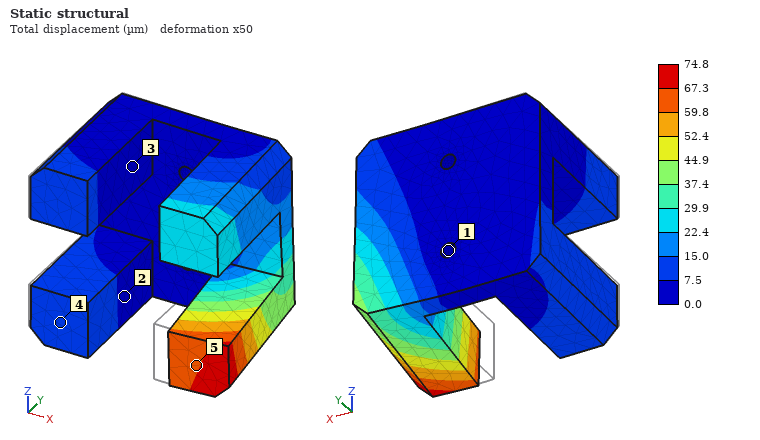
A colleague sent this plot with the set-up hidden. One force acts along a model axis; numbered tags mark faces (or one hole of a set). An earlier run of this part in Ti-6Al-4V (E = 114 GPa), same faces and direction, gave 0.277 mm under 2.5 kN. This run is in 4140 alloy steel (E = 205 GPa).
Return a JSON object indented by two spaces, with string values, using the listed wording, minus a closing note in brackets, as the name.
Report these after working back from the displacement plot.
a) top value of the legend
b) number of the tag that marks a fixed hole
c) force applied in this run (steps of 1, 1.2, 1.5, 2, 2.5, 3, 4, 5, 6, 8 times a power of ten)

{
  "top value of the legend": "74.8 µm",
  "number of the tag that marks a fixed hole": "1",
  "force applied in this run": "1.2 kN"
}
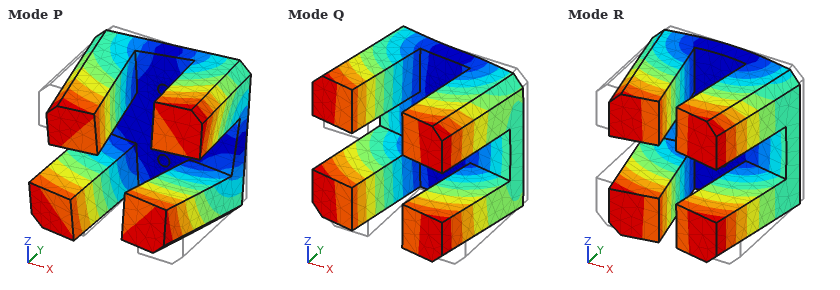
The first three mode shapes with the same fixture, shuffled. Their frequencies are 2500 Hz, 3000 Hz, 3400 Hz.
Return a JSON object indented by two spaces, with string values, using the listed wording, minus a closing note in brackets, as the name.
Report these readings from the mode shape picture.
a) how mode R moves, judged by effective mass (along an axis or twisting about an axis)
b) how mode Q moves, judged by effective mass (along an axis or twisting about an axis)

{
  "how mode R moves, judged by effective mass": "along Y",
  "how mode Q moves, judged by effective mass": "along X"
}
